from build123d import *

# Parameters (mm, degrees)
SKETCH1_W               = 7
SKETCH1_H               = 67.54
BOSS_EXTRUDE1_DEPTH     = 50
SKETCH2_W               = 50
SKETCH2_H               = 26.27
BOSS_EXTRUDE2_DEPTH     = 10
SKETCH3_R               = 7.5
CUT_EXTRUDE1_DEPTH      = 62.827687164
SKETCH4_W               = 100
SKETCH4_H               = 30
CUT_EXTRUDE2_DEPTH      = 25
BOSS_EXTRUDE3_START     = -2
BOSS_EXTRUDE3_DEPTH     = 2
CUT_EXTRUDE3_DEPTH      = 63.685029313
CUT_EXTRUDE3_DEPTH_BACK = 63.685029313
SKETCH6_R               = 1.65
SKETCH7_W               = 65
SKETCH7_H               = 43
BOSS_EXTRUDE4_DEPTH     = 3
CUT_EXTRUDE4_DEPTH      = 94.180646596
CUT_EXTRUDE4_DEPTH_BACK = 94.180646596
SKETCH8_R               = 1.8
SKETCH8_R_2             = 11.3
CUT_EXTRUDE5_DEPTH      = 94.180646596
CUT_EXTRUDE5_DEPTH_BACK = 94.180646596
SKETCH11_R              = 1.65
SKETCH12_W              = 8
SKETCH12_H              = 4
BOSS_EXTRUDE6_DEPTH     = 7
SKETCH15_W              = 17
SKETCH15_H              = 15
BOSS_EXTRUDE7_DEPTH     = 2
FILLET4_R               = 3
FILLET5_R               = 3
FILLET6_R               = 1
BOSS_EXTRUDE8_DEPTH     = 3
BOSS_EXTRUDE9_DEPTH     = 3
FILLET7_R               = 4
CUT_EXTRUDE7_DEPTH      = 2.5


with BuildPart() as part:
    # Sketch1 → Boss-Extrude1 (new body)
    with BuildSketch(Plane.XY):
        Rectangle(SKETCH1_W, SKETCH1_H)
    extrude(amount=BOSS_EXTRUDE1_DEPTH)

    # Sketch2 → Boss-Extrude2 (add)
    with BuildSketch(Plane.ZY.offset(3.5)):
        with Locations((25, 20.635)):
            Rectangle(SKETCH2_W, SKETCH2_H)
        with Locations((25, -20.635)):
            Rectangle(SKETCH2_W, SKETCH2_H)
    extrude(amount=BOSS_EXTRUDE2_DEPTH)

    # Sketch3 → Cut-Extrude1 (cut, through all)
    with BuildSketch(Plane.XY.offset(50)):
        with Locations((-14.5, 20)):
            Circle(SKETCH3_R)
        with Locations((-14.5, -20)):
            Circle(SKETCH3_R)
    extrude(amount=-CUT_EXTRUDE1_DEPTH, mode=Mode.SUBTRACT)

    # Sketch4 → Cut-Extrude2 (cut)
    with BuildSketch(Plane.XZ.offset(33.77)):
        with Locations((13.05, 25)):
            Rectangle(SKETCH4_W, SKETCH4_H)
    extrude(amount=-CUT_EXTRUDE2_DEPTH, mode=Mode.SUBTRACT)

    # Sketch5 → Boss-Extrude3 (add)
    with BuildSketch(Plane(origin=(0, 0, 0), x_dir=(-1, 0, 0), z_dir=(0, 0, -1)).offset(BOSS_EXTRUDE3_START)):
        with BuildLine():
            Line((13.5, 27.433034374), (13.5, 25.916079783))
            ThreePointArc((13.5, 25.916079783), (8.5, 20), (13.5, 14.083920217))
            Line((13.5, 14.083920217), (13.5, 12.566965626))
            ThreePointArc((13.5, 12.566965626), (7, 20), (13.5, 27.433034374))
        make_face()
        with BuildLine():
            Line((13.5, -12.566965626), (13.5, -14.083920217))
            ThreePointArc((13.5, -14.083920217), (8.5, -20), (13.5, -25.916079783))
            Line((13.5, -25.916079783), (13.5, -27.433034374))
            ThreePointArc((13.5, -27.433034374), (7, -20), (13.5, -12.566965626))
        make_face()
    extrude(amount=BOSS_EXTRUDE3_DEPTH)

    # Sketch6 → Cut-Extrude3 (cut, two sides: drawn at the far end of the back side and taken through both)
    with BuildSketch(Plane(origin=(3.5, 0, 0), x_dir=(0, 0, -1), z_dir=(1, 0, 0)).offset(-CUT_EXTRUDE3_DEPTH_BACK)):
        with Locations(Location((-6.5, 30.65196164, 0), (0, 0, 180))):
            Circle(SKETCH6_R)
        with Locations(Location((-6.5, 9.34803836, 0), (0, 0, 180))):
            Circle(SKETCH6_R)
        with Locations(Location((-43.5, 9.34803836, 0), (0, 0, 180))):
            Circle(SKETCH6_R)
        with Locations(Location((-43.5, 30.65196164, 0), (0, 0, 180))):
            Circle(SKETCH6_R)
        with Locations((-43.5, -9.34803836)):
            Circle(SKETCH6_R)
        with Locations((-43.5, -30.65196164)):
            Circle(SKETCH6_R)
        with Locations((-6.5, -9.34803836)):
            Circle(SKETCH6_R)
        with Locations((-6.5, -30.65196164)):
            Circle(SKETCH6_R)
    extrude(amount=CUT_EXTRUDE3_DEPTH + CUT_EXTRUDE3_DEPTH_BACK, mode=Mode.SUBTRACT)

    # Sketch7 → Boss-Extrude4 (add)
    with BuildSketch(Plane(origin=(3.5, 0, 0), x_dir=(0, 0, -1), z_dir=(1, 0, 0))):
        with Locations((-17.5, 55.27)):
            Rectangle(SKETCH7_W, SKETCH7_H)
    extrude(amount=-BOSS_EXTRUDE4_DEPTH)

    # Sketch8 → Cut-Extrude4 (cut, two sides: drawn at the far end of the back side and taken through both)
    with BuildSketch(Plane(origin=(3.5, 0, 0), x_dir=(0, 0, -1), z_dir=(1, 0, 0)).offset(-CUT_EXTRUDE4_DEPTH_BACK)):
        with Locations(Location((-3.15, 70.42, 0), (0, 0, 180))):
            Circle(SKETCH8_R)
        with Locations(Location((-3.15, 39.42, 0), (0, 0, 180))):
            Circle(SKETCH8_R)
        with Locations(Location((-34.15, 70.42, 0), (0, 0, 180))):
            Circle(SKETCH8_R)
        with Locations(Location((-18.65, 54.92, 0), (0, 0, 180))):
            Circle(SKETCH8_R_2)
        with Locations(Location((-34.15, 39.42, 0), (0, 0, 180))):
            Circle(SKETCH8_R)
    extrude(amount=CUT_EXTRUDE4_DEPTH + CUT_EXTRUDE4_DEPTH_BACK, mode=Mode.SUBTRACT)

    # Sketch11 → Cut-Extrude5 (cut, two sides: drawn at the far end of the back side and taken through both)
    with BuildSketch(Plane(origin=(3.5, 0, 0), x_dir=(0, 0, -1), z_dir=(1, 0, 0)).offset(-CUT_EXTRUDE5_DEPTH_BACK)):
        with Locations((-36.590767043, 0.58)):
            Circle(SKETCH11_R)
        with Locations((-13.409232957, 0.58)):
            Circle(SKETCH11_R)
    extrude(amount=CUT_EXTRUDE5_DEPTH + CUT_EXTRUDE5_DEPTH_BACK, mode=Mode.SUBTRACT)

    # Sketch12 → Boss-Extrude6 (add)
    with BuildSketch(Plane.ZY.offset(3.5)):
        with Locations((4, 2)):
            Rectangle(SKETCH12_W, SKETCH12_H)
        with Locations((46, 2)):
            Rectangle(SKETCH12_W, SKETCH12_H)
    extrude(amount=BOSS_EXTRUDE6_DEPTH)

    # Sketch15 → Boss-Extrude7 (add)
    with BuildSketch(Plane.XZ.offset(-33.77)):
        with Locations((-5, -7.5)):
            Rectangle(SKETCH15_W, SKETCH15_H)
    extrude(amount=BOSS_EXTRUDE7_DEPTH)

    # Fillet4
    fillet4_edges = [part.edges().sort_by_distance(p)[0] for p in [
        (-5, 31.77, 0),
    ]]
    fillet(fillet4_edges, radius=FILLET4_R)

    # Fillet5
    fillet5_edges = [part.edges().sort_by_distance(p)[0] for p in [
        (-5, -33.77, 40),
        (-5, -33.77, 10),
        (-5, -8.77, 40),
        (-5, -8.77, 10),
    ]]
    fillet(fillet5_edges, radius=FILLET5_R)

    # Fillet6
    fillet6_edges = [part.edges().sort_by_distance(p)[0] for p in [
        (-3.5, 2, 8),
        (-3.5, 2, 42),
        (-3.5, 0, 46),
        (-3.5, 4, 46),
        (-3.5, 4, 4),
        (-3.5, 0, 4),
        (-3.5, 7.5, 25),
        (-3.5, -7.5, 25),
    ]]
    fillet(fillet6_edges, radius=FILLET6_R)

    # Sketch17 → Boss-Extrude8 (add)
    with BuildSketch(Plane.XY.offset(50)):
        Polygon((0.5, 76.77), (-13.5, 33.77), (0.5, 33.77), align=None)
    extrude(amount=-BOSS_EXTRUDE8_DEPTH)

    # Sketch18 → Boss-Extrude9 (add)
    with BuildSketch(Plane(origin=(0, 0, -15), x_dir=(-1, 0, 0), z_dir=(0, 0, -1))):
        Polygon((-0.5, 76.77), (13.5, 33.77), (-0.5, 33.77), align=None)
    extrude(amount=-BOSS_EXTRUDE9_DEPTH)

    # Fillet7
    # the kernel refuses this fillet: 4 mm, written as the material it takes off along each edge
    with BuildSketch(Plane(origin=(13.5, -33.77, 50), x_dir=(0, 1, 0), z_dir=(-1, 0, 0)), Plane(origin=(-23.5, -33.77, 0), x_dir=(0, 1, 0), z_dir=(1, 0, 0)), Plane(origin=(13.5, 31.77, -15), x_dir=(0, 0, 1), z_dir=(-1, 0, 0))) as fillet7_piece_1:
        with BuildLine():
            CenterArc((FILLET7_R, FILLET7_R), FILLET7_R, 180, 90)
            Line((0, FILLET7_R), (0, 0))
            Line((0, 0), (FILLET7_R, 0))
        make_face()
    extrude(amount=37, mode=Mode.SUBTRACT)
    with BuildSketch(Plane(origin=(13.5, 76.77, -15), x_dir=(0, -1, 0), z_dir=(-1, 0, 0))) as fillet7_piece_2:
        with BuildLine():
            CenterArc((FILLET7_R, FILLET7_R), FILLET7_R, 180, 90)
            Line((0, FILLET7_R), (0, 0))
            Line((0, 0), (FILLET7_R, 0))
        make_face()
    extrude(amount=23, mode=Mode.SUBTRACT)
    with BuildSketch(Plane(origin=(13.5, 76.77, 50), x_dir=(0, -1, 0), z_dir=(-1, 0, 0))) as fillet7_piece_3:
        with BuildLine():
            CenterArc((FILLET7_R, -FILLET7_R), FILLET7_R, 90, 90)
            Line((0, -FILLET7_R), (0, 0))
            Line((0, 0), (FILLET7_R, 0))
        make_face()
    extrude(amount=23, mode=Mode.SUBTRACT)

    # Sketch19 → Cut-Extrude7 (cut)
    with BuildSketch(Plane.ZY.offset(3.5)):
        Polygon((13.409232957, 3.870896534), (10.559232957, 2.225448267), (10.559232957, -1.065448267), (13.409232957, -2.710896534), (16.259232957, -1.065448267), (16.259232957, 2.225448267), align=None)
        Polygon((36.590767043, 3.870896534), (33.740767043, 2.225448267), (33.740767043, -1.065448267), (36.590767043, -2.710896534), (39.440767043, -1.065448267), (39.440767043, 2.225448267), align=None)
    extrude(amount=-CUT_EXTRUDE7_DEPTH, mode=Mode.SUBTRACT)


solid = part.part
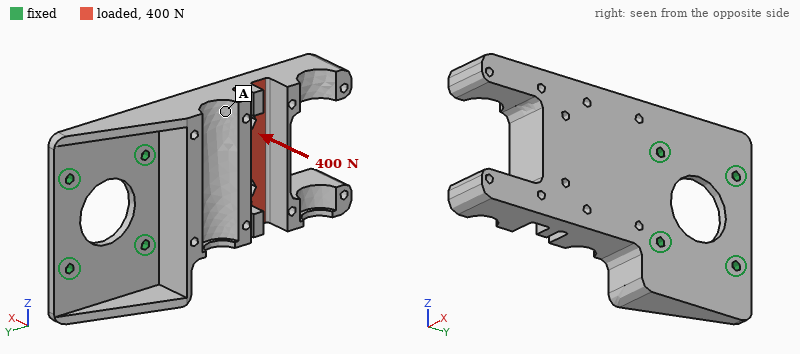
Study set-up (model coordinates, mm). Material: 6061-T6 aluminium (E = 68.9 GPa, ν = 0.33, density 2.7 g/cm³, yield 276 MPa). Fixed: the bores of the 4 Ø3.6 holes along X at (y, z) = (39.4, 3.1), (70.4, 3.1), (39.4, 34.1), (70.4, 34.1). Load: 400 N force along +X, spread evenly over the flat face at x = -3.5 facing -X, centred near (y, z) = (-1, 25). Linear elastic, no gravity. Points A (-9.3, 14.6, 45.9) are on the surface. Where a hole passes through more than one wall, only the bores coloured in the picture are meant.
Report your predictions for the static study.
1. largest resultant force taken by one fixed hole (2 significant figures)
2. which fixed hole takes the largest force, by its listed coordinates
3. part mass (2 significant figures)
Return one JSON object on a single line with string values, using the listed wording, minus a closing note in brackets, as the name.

{"largest resultant force taken by one fixed hole": "760 N", "which fixed hole takes the largest force, by its listed coordinates": "(39.4, 34.1)", "part mass": "110 g"}
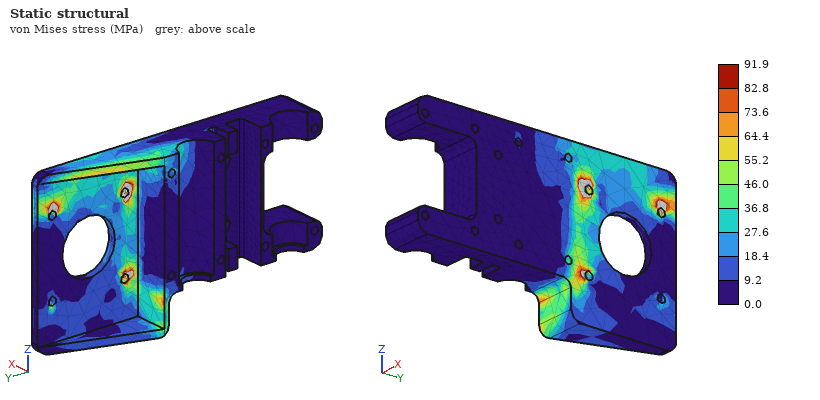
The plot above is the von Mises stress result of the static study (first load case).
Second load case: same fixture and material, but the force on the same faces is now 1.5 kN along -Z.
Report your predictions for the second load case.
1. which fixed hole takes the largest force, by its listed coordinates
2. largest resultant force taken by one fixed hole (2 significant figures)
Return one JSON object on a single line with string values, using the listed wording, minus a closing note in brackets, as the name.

{"which fixed hole takes the largest force, by its listed coordinates": "(39.4, 3.1)", "largest resultant force taken by one fixed hole": "1.7 kN"}
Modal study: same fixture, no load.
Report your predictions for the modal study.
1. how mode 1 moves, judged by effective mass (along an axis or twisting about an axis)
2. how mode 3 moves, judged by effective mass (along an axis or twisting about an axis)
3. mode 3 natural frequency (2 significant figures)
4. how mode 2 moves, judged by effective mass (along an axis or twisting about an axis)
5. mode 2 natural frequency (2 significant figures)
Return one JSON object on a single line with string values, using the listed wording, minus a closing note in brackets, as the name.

{"how mode 1 moves, judged by effective mass": "along X", "how mode 3 moves, judged by effective mass": "along Z", "mode 3 natural frequency": "4100 Hz", "how mode 2 moves, judged by effective mass": "twisting about Y", "mode 2 natural frequency": "2400 Hz"}
